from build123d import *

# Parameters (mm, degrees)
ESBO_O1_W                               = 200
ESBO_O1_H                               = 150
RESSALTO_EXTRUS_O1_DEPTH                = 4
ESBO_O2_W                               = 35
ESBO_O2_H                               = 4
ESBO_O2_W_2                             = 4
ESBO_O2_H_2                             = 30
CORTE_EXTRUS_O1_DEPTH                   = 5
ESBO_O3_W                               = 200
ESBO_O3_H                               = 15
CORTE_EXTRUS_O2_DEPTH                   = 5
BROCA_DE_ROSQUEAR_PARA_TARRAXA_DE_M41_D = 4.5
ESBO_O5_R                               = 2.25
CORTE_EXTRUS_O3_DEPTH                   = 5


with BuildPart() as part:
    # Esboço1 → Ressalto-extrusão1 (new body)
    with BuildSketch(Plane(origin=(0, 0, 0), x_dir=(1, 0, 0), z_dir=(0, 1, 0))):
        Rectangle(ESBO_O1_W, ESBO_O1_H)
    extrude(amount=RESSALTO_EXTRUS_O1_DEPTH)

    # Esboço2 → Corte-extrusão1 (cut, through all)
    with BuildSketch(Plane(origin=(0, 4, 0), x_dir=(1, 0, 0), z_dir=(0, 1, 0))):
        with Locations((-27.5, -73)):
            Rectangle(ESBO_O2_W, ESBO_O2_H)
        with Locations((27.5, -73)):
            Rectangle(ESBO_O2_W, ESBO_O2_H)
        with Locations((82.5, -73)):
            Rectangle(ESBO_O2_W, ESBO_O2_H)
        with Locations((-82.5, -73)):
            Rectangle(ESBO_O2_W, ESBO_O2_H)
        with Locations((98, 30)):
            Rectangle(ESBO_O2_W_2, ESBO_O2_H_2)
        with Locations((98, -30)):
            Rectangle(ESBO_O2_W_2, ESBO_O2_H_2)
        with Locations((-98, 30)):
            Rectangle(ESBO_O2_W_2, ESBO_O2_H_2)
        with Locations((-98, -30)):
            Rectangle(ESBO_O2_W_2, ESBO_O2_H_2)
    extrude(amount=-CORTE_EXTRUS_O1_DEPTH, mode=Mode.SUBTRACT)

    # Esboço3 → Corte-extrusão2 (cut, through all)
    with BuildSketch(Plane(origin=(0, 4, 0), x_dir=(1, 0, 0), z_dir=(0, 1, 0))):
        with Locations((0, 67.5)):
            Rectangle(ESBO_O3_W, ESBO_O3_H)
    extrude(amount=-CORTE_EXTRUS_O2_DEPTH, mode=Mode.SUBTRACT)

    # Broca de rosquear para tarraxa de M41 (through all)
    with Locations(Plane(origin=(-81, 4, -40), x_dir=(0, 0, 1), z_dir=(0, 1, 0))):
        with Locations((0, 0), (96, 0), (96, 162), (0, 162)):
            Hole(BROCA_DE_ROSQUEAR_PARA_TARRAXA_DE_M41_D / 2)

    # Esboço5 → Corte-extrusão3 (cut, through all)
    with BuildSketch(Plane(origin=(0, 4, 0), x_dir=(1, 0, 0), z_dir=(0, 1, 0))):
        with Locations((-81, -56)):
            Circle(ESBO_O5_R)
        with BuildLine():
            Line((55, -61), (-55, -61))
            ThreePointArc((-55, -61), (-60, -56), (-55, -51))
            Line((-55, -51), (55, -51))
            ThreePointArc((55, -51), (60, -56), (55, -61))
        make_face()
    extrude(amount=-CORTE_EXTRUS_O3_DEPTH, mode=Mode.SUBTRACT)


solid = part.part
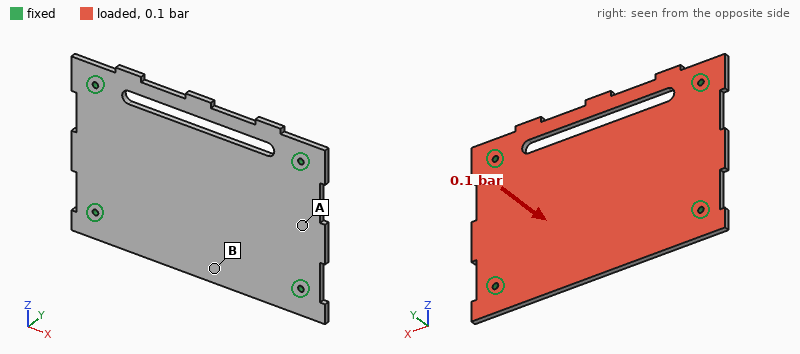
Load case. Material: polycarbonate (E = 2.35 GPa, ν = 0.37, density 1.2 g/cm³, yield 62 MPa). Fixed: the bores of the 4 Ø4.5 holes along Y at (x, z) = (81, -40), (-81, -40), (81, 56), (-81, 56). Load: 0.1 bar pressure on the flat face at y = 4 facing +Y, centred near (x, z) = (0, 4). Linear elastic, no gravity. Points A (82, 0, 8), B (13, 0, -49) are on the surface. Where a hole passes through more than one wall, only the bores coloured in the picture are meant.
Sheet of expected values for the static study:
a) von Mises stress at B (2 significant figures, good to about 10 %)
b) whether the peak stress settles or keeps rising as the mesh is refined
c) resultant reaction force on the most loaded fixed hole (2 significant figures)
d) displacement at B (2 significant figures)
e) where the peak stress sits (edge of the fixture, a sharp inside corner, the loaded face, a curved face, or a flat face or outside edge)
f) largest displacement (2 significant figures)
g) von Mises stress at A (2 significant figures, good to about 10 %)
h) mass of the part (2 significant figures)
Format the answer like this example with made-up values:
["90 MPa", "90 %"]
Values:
["4.5 MPa", "keeps rising", "66 N", "1.8 mm", "edge of the fixture", "2.1 mm", "2.1 MPa", "120 g"]
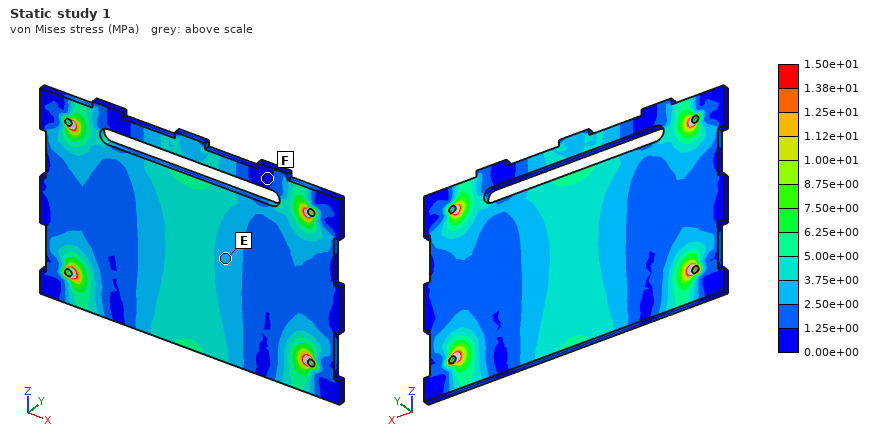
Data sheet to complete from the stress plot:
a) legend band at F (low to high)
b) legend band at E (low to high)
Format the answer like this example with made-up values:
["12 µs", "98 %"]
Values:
["0.00e+00 to 1.25e+00 MPa", "2.50e+00 to 3.75e+00 MPa"]
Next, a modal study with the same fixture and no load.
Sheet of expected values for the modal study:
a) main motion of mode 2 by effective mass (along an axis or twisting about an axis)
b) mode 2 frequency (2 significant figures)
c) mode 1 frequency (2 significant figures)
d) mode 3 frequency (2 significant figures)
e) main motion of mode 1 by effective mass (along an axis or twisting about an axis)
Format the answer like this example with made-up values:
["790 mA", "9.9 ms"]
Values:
["twisting about X", "260 Hz", "190 Hz", "310 Hz", "along Y"]
